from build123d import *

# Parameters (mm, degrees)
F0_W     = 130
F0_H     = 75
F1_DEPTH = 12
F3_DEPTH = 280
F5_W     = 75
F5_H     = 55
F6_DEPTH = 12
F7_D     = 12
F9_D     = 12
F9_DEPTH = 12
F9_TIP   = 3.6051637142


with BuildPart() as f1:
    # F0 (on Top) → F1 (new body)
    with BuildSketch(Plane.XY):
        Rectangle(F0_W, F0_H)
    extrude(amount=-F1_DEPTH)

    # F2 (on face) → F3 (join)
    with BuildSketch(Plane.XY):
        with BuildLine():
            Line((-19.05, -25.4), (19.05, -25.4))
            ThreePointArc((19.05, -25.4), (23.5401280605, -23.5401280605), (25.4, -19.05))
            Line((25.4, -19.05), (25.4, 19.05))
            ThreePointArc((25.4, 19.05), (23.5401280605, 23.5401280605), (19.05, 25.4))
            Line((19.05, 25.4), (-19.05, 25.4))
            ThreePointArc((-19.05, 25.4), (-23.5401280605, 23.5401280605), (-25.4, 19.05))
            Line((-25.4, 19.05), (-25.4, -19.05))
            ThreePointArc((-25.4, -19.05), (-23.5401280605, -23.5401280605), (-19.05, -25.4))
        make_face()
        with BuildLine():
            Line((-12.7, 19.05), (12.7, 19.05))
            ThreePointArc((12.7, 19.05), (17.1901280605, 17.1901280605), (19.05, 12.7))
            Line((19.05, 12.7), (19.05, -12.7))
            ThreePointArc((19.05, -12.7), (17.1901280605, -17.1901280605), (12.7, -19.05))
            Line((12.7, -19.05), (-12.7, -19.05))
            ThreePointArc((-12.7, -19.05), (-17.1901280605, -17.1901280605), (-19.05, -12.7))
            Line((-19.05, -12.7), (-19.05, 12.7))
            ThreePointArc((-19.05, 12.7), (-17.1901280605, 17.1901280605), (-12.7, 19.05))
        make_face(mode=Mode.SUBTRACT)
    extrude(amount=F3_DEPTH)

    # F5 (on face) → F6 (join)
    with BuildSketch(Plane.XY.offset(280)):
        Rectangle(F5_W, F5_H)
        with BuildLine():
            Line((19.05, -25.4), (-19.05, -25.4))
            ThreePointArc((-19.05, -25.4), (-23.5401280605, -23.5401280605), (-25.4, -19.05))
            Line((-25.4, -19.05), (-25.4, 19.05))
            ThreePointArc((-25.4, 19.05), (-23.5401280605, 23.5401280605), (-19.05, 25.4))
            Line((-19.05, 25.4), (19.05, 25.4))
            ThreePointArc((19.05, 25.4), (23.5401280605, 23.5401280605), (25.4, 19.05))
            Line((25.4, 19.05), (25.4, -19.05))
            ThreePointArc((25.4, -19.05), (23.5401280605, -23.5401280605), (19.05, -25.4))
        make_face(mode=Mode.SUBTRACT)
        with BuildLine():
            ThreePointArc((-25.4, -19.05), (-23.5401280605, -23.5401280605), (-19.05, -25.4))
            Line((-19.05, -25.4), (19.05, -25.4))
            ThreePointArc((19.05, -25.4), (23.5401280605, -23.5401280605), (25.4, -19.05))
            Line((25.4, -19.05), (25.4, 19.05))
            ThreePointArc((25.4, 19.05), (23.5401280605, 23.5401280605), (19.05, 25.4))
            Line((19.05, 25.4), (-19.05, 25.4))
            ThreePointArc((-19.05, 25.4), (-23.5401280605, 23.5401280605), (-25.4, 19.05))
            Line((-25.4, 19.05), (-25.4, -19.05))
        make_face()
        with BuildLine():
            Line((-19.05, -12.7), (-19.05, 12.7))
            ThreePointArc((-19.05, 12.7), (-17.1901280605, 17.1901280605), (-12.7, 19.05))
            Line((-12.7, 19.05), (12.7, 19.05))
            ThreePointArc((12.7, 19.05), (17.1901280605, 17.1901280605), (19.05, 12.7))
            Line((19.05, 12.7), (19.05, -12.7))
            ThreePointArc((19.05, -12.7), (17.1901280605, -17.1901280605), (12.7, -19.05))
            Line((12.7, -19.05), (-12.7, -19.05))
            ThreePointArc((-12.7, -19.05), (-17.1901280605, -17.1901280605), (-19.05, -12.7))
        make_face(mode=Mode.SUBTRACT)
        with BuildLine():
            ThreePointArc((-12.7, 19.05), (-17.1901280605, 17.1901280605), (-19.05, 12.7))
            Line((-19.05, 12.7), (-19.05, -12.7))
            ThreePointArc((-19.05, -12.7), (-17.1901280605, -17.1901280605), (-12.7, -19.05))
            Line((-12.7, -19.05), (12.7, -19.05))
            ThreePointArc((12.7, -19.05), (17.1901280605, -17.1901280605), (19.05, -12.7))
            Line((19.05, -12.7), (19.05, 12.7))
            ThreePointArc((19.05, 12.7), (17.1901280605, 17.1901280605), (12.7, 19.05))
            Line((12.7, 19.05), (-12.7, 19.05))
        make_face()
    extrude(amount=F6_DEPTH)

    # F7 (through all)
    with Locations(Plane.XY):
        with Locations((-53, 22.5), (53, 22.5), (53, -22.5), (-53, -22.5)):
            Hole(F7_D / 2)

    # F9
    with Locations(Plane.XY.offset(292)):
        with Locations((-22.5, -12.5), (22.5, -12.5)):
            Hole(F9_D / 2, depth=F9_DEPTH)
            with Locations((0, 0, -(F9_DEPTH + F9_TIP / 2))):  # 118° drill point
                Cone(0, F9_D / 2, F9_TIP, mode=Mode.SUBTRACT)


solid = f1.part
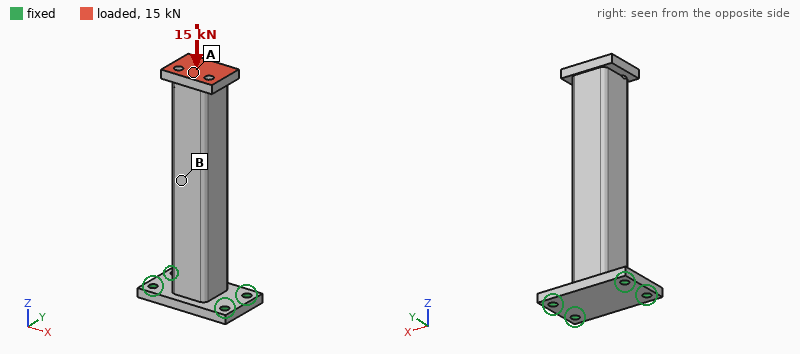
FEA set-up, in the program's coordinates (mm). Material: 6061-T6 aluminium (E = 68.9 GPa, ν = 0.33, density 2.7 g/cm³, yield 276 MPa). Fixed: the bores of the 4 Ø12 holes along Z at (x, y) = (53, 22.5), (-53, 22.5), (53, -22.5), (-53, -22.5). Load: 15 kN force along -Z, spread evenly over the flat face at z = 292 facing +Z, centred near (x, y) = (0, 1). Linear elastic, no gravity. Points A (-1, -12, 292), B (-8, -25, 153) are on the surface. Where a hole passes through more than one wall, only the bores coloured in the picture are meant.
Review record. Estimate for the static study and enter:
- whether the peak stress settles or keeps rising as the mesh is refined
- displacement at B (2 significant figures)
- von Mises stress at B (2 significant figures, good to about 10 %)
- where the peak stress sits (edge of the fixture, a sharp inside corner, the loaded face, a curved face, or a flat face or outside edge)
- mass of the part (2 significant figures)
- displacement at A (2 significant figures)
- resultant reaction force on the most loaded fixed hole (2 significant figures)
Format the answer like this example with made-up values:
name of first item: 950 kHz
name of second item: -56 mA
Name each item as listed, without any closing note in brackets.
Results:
whether the peak stress settles or keeps rising as the mesh is refined: keeps rising
displacement at B: 0.074 mm
von Mises stress at B: 13 MPa
where the peak stress sits: edge of the fixture
mass of the part: 1.3 kg
displacement at A: 0.11 mm
resultant reaction force on the most loaded fixed hole: 4.0 kN
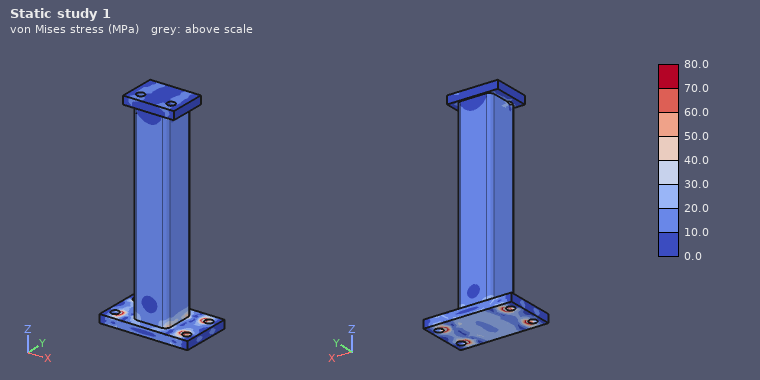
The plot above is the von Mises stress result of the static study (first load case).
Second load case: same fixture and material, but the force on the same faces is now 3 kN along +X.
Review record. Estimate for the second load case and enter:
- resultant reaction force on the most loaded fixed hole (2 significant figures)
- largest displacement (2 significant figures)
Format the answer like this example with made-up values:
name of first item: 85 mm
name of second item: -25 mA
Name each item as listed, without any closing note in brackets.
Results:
resultant reaction force on the most loaded fixed hole: 5.9 kN
largest displacement: 1.6 mm
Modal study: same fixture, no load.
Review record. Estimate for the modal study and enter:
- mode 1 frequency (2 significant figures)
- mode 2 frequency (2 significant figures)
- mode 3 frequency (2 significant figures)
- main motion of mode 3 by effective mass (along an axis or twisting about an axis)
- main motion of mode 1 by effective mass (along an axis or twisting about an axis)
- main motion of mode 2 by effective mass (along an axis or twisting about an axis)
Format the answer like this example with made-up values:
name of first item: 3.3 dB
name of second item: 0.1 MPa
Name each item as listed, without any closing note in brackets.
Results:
mode 1 frequency: 300 Hz
mode 2 frequency: 380 Hz
mode 3 frequency: 2100 Hz
main motion of mode 3 by effective mass: twisting about Z
main motion of mode 1 by effective mass: along Y
main motion of mode 2 by effective mass: along X
